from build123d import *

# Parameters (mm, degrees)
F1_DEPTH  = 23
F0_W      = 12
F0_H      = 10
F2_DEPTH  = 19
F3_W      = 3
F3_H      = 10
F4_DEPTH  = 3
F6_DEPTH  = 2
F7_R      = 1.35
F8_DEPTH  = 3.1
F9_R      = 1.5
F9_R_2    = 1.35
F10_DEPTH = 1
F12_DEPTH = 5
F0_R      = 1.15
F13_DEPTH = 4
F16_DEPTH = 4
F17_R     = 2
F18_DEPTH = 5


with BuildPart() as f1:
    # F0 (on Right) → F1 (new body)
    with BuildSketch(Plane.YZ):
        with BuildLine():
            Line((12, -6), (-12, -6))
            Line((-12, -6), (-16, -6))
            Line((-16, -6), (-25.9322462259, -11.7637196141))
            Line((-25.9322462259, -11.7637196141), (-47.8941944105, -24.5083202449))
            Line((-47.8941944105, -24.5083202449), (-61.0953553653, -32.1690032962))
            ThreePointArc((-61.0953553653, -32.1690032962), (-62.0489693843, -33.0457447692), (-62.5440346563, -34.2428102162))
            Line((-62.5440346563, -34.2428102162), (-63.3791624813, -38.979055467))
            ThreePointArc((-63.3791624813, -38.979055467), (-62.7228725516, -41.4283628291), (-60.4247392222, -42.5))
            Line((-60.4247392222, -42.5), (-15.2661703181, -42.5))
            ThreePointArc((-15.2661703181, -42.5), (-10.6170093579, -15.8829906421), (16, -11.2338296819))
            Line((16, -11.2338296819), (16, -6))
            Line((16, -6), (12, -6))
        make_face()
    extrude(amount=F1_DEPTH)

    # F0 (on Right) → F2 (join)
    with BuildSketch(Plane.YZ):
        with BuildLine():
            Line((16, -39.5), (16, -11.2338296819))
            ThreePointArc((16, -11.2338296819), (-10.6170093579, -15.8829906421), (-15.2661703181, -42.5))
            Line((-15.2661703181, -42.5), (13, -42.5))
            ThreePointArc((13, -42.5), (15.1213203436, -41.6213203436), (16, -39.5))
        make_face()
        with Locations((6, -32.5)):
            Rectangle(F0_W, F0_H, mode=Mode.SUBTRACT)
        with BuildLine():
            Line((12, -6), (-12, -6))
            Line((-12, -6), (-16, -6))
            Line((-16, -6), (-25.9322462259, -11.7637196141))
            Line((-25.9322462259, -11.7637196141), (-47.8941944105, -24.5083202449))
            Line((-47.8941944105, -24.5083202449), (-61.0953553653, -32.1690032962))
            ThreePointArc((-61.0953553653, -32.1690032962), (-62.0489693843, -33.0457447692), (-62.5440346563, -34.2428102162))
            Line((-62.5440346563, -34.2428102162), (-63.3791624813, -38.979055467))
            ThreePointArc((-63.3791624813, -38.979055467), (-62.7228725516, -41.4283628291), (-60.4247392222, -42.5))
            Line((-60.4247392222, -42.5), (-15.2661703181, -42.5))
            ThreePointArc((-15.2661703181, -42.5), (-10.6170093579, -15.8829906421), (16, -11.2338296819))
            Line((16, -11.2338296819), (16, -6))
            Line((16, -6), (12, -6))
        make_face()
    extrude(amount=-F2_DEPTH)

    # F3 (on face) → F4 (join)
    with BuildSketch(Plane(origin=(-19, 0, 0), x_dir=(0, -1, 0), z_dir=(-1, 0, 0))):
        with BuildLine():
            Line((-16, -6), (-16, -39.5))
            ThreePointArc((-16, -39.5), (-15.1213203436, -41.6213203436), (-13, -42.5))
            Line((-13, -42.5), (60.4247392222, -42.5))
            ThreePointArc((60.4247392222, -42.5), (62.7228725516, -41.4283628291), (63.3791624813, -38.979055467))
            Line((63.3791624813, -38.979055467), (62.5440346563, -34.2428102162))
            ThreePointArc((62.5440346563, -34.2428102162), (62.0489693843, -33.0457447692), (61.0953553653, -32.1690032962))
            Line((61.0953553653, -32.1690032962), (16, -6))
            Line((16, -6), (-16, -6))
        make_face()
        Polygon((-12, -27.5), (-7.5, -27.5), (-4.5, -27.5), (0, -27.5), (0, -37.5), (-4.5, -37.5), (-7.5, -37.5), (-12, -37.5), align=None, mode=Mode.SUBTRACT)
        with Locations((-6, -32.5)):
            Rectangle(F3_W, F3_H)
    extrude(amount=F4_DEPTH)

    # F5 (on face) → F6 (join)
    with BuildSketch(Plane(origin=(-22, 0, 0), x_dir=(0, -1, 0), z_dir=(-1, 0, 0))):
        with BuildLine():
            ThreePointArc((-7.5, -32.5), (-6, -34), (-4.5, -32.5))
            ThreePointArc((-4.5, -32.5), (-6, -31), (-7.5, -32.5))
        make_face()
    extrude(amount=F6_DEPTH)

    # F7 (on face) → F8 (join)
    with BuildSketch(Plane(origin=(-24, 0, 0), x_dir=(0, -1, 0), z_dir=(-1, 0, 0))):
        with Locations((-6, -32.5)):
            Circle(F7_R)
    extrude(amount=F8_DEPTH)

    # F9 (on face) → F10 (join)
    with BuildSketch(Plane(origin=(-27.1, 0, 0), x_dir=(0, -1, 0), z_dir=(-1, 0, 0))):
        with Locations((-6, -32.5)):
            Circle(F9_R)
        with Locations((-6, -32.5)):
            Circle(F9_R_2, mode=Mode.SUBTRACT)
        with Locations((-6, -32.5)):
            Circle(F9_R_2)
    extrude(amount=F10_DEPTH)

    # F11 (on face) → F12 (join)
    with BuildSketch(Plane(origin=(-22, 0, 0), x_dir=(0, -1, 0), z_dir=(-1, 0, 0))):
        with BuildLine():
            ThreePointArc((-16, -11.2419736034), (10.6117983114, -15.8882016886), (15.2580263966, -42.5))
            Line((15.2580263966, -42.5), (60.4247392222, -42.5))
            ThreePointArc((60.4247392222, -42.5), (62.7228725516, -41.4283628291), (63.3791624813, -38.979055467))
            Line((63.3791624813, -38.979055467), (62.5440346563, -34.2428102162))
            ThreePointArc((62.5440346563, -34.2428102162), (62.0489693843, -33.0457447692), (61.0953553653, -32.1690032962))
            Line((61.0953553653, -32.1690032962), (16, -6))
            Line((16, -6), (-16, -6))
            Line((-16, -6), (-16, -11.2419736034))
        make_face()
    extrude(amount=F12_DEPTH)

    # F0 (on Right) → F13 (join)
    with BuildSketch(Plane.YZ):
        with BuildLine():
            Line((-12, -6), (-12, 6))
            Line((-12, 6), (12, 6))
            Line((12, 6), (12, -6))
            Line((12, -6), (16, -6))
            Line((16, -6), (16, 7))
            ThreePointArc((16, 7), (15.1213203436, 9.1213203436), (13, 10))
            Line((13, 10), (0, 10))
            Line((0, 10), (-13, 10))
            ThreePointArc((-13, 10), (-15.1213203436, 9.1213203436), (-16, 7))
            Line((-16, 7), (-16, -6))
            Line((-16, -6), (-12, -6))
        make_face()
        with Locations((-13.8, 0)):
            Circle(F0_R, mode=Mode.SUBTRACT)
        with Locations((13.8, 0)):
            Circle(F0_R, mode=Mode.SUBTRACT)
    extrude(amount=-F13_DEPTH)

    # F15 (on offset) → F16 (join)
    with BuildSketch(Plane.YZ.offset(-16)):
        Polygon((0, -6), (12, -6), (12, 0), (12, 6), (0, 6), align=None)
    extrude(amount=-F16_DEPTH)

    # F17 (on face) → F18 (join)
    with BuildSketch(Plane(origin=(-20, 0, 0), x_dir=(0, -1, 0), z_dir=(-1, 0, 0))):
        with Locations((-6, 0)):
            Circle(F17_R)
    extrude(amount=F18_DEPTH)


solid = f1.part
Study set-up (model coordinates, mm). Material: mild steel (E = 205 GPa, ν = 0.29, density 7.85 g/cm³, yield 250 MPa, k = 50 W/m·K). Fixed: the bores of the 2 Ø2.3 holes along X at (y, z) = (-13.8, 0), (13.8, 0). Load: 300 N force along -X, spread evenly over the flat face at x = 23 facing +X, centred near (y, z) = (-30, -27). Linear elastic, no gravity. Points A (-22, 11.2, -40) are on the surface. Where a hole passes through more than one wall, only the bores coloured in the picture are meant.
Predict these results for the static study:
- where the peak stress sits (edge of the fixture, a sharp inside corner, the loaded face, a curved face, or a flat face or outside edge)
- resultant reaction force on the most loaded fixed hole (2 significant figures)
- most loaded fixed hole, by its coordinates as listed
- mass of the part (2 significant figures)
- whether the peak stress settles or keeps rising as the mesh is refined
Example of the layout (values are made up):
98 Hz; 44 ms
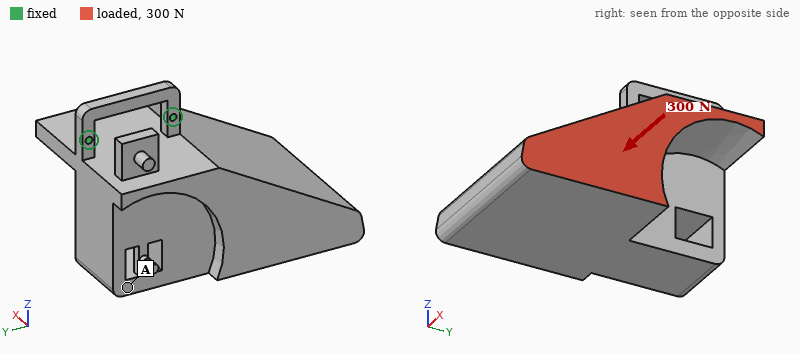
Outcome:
edge of the fixture; 460 N; (-13.8, 0); 650 g; keeps rising
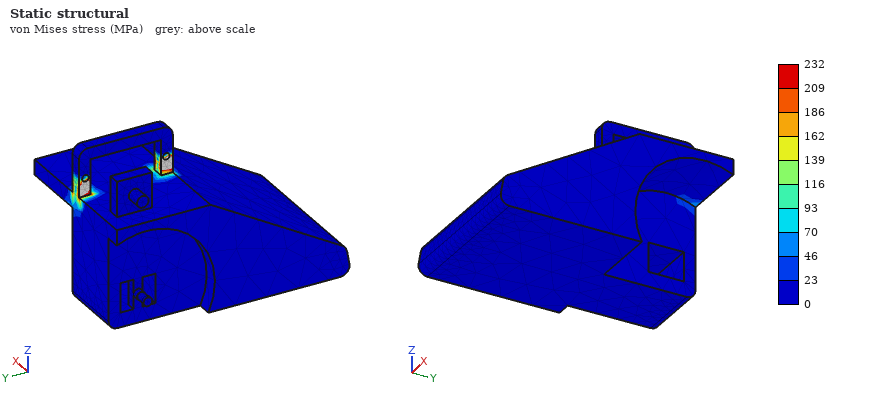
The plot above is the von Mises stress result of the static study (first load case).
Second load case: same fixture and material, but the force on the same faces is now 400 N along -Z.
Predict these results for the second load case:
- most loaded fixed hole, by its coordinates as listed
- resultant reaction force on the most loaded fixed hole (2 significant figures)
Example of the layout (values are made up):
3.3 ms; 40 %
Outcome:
(-13.8, 0); 630 N
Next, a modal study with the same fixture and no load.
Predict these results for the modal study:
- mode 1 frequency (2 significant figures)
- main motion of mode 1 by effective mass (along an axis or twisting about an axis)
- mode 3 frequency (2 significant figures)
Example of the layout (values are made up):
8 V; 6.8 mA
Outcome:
250 Hz; along X; 1600 Hz
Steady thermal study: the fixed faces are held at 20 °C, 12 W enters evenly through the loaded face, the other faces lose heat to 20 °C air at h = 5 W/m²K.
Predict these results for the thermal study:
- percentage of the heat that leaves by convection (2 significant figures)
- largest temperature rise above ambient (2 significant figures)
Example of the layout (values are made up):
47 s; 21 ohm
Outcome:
26 %; 49 K
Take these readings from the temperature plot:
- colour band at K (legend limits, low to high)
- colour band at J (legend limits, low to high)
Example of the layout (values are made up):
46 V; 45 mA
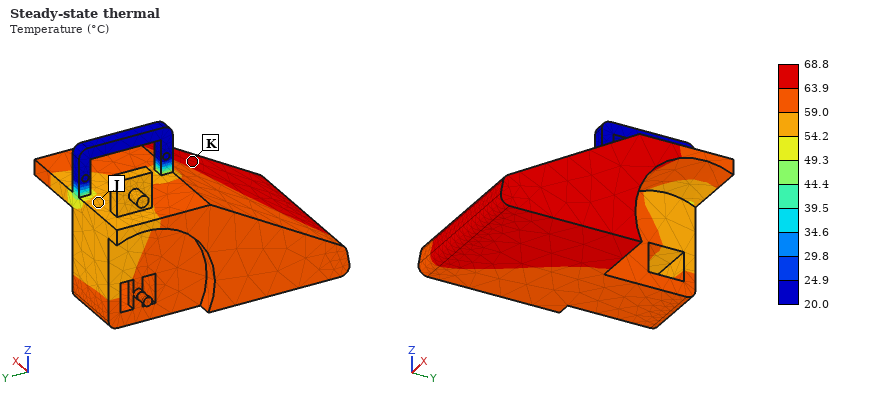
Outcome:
63.9 to 68.8 °C; 54.2 to 59.0 °C
